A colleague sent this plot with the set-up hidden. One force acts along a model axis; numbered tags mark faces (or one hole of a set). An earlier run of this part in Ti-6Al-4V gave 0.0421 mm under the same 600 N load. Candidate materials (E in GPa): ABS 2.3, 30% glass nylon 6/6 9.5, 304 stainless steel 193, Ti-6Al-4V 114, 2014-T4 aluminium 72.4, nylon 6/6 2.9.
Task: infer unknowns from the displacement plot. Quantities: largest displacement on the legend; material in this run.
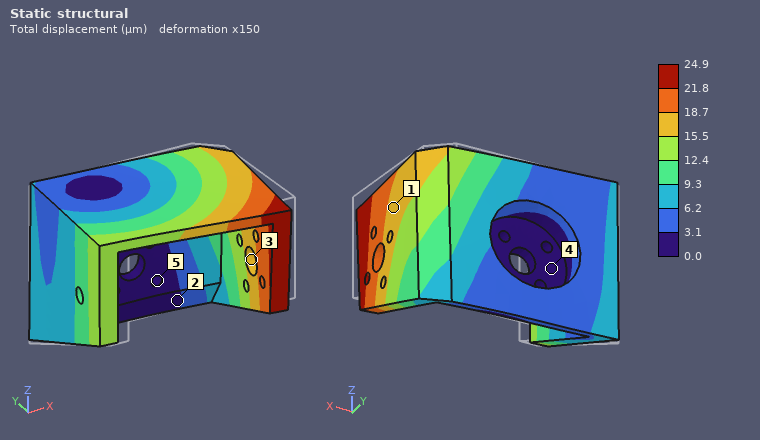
24.9 µm
304 stainless steel
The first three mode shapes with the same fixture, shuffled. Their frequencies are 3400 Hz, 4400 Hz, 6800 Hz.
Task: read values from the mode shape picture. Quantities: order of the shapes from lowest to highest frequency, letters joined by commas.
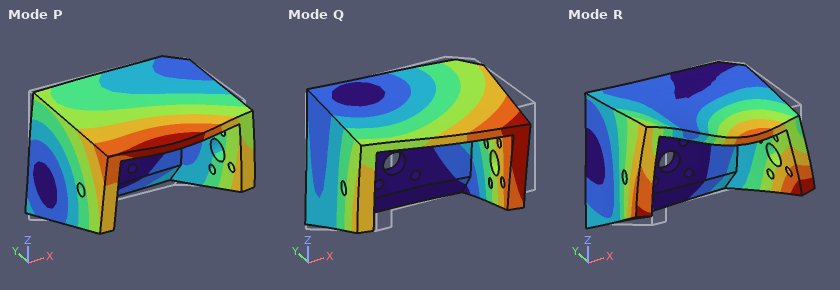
Q, P, R
